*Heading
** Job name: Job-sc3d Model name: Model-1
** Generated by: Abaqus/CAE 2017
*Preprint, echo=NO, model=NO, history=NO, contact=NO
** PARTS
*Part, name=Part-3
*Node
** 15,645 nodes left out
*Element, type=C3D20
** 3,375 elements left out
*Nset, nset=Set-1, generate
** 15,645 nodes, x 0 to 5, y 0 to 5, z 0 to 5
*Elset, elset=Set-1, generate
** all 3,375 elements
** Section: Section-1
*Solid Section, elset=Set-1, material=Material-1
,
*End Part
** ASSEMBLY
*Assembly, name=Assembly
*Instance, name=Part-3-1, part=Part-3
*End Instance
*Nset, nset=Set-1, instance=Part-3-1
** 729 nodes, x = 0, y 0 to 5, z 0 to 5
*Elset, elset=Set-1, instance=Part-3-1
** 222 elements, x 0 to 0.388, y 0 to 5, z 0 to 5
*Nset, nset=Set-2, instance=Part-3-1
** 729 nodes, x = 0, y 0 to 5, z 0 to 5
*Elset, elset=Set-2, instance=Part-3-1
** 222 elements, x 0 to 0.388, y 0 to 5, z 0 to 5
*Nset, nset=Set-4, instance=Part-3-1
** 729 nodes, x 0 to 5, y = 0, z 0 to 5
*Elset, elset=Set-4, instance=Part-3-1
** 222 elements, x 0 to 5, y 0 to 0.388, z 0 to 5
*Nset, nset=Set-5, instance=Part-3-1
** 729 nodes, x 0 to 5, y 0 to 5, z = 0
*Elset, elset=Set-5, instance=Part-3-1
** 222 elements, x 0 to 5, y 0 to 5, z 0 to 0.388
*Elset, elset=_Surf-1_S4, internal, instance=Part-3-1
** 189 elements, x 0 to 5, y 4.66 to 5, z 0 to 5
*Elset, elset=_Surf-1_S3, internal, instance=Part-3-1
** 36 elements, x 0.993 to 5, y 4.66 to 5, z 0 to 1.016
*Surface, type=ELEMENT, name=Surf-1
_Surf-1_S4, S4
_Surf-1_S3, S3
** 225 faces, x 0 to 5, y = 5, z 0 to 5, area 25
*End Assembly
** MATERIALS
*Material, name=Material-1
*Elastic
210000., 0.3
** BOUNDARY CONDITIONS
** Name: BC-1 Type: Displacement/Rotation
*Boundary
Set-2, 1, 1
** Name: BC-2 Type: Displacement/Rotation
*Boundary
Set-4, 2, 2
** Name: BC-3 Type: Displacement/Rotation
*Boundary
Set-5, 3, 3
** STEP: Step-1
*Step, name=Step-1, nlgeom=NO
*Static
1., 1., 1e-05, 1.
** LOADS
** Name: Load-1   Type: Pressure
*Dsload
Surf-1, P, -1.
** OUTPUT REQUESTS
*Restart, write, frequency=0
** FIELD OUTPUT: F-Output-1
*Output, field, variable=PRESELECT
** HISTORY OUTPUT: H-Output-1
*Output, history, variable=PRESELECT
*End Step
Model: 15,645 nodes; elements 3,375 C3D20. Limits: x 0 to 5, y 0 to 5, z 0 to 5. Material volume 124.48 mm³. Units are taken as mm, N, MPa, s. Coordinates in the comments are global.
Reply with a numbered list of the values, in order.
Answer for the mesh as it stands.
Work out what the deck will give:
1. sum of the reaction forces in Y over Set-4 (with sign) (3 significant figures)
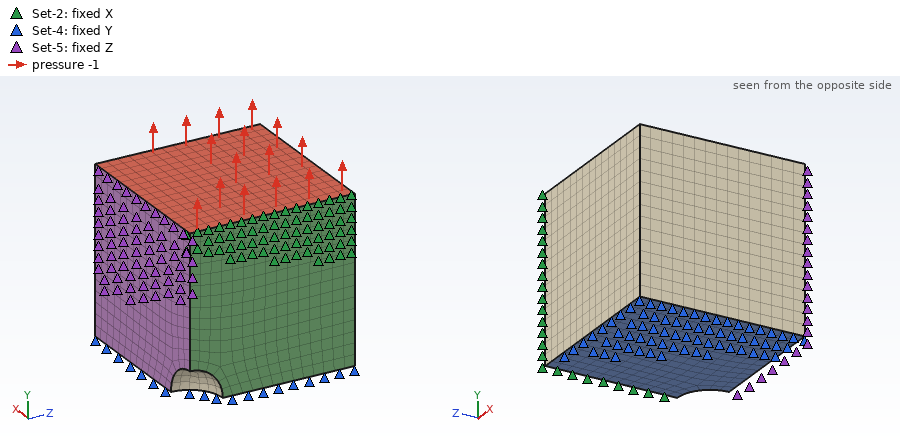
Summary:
1. -25.0 N
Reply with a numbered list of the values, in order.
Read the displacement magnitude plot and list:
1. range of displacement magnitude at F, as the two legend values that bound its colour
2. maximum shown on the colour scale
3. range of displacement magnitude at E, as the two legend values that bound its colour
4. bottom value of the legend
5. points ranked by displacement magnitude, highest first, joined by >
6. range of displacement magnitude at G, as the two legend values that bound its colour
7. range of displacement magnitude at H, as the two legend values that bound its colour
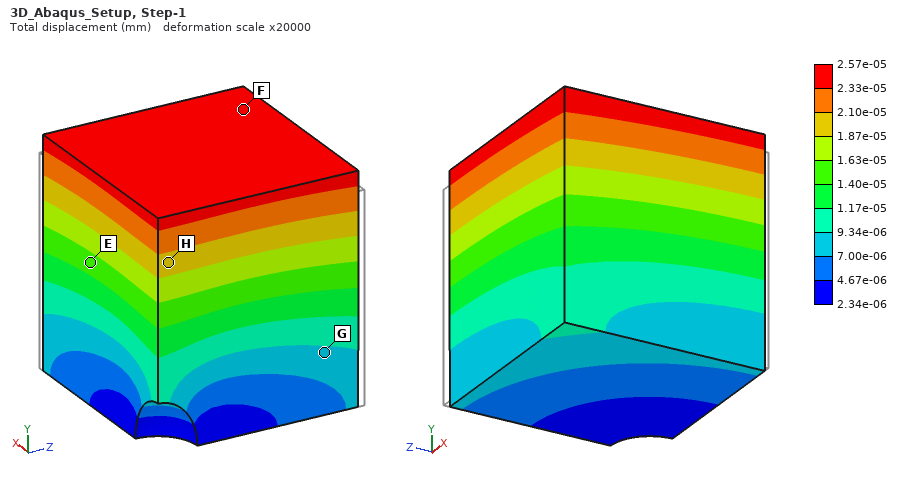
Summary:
1. 2.33e-05 to 2.57e-05 mm
2. 2.57e-05 mm
3. 1.40e-05 to 1.63e-05 mm
4. 2.34e-06 mm
5. F > H > E > G
6. 7.00e-06 to 9.34e-06 mm
7. 1.87e-05 to 2.10e-05 mm
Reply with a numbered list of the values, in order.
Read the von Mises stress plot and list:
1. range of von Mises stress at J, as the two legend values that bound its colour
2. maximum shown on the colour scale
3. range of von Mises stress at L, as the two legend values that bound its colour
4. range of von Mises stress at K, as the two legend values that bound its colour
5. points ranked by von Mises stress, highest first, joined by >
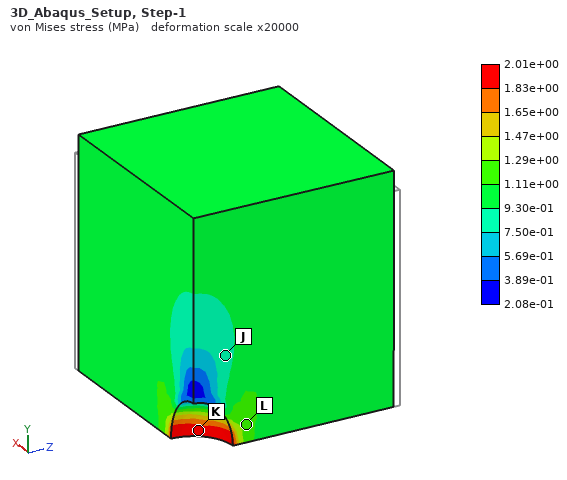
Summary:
1. 7.50e-01 to 9.30e-01 MPa
2. 2.01e+00 MPa
3. 1.11e+00 to 1.29e+00 MPa
4. 1.83e+00 to 2.01e+00 MPa
5. K > L > J
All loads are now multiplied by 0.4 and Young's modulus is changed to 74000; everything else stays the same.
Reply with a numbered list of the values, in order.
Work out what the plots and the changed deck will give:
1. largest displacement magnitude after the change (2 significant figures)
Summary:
1. 2.9e-05 mm
